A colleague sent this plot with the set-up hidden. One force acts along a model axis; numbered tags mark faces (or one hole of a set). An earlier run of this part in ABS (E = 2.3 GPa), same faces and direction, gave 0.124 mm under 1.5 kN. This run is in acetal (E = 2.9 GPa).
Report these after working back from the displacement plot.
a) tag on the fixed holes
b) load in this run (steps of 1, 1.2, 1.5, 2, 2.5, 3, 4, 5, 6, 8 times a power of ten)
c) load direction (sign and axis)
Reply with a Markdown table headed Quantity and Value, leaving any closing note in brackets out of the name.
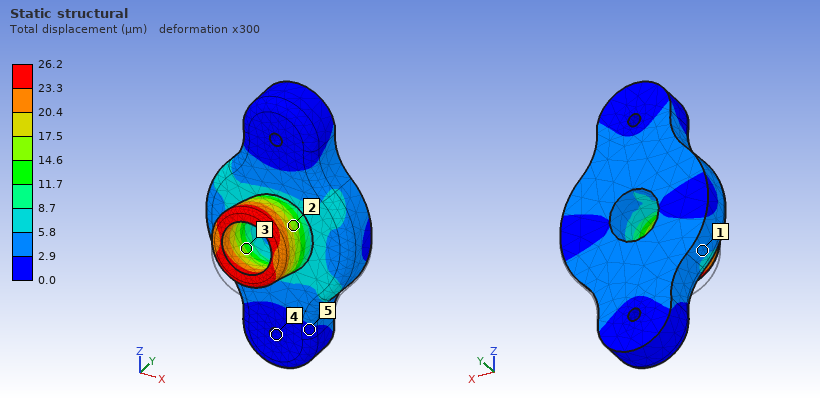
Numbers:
| Quantity | Value |
|---|---|
| tag on the fixed holes | 4 |
| load in this run | 400 N |
| load direction | +Z |
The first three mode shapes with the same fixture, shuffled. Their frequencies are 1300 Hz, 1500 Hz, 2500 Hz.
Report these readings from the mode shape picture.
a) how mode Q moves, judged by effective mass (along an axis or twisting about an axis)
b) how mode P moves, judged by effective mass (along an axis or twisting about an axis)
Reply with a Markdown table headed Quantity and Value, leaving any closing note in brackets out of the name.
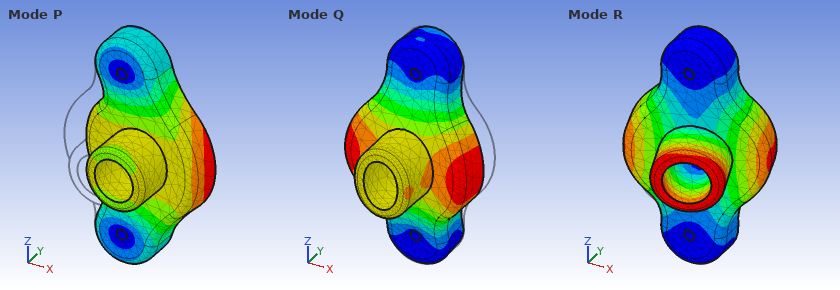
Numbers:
| Quantity | Value |
|---|---|
| how mode Q moves, judged by effective mass | along Y |
| how mode P moves, judged by effective mass | along X |
